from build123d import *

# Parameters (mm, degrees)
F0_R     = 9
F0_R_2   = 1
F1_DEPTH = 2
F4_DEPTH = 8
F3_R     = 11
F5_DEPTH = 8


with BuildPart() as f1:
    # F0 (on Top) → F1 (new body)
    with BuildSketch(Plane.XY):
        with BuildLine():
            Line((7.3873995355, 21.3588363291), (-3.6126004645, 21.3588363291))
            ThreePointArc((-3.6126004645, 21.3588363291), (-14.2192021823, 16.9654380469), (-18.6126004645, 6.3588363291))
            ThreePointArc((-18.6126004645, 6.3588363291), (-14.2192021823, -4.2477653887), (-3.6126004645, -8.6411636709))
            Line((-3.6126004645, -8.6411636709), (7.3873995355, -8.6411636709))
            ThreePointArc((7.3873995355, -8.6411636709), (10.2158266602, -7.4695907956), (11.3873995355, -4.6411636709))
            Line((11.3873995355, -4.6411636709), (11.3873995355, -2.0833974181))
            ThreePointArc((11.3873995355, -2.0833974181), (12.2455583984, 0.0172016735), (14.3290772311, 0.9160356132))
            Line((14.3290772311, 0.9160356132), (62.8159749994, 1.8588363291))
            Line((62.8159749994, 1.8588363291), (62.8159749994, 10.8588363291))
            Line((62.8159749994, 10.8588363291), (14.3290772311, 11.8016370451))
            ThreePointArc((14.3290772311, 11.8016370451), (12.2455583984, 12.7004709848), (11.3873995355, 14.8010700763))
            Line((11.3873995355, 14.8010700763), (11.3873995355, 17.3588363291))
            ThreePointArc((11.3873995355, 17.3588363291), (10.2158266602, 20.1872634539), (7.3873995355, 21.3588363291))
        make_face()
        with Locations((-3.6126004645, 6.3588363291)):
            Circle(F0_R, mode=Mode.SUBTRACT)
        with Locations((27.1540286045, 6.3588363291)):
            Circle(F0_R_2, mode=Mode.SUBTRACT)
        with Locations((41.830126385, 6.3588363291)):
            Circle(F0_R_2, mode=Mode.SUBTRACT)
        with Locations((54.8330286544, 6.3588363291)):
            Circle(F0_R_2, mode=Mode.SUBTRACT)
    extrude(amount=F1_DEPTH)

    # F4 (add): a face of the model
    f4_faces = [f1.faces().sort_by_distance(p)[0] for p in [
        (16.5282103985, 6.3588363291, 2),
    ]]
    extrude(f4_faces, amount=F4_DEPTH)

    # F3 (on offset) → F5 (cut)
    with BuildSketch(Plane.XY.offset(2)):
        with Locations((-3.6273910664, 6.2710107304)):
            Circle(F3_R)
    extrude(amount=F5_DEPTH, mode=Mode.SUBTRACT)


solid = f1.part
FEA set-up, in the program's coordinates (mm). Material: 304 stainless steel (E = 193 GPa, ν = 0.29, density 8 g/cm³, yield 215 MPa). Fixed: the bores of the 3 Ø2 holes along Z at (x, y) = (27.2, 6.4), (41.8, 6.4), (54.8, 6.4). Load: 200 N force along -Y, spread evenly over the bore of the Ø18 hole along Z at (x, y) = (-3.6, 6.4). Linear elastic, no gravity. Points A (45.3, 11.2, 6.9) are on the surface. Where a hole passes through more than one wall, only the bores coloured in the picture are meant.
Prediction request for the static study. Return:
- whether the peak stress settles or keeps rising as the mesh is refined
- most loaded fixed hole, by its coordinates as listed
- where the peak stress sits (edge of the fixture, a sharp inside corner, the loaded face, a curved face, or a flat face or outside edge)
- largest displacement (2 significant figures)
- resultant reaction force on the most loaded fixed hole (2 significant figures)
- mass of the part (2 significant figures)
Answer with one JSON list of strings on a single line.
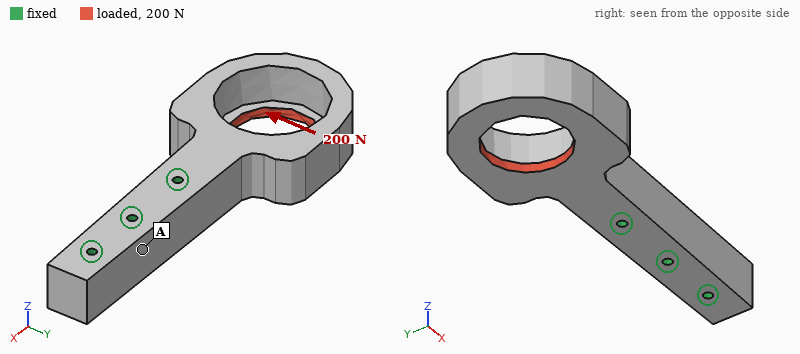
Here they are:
["keeps rising", "(27.2, 6.4)", "edge of the fixture", "29 µm", "520 N", "76 g"]
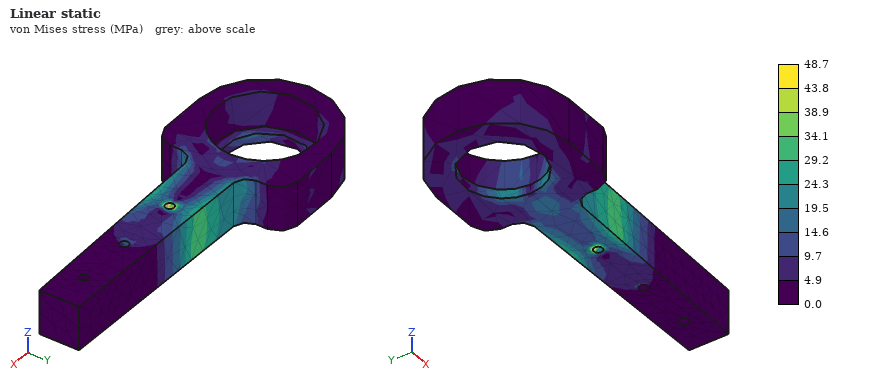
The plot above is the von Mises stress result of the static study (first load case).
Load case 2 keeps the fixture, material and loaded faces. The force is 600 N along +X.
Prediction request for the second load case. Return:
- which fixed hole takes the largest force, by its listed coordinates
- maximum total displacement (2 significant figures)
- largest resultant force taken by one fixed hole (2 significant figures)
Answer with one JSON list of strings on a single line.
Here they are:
["(27.2, 6.4)", "15 µm", "520 N"]
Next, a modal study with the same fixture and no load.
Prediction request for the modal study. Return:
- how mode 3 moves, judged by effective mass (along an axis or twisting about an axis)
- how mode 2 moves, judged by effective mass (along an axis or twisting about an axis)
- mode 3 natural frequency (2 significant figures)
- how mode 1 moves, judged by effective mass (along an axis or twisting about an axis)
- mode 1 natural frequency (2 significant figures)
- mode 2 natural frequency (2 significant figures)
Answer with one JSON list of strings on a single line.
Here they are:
["twisting about X", "along Z", "6200 Hz", "along Y", "2700 Hz", "3100 Hz"]
